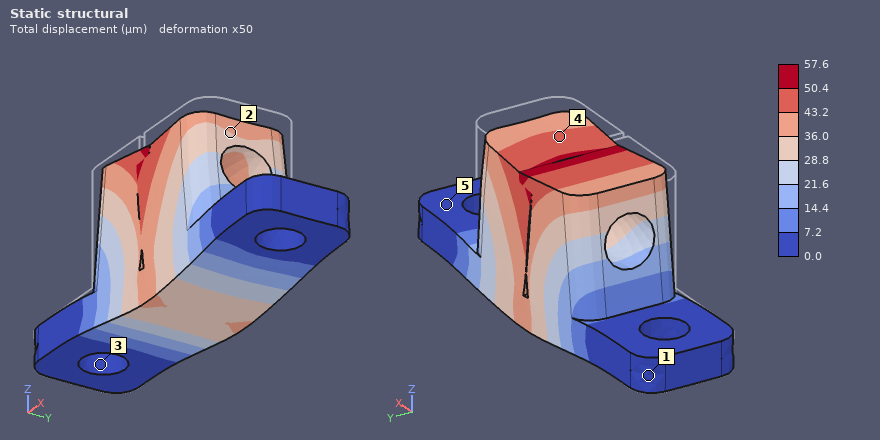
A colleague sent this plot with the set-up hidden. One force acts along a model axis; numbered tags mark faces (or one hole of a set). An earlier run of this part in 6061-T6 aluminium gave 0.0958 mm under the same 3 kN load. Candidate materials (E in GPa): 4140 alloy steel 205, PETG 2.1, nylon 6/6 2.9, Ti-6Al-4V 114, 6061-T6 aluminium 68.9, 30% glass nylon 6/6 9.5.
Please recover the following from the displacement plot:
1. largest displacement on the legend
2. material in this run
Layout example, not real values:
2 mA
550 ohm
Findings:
57.6 µm
Ti-6Al-4V
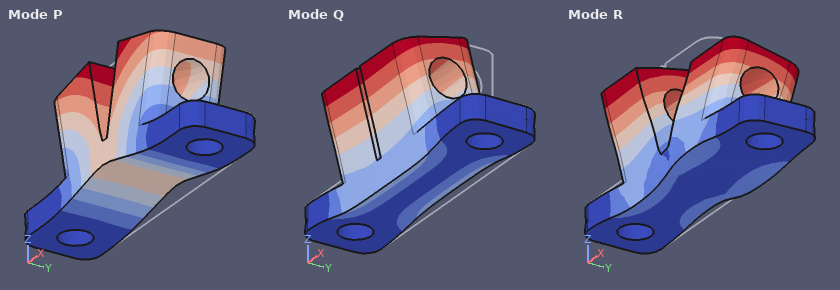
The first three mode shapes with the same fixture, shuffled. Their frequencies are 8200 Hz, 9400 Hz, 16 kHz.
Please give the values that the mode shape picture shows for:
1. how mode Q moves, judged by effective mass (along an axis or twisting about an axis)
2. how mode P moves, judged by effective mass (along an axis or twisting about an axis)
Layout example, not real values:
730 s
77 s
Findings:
along Y
along Z
